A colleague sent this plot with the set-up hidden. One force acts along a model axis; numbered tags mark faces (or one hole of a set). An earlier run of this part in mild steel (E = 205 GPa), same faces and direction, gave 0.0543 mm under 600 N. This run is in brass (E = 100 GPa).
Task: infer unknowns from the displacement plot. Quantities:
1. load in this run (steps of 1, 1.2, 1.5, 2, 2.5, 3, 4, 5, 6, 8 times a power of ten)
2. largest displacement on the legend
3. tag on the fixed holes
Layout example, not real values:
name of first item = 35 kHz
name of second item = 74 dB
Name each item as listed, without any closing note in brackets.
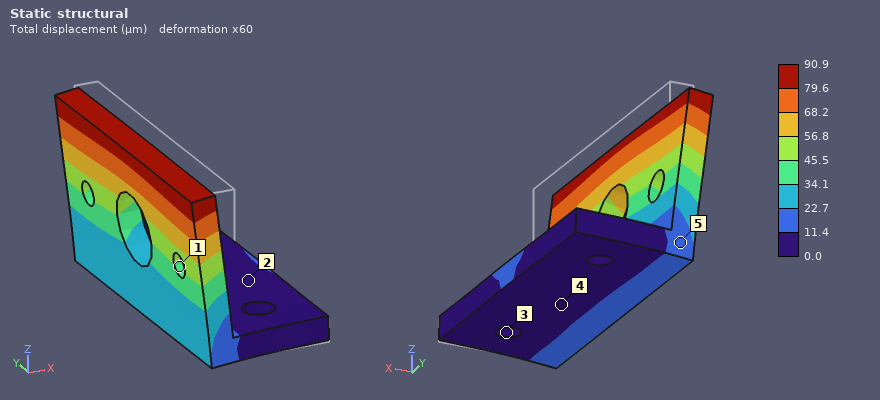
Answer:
load in this run = 500 N
largest displacement on the legend = 90.9 µm
tag on the fixed holes = 3
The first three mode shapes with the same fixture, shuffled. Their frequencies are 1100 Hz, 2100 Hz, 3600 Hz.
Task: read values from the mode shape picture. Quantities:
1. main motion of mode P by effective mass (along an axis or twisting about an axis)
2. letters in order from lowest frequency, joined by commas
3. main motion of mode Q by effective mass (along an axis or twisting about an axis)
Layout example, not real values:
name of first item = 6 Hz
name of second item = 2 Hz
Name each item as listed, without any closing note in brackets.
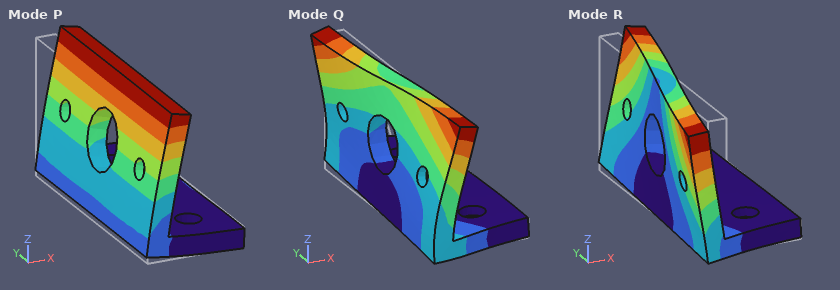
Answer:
main motion of mode P by effective mass = along X
letters in order from lowest frequency, joined by commas = P, R, Q
main motion of mode Q by effective mass = along Y
